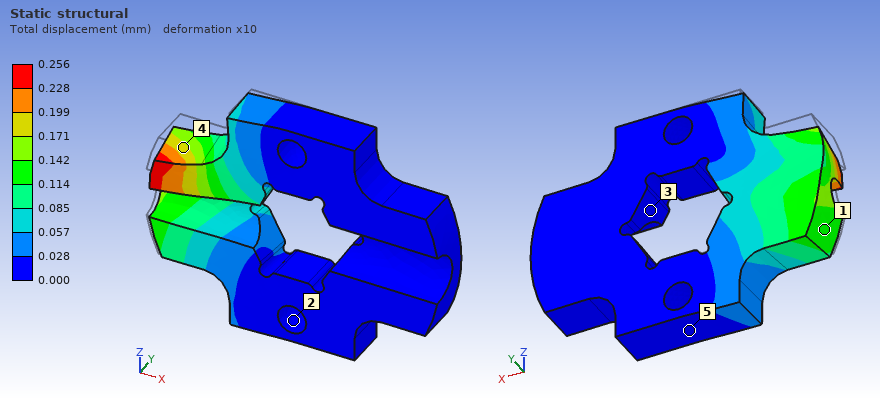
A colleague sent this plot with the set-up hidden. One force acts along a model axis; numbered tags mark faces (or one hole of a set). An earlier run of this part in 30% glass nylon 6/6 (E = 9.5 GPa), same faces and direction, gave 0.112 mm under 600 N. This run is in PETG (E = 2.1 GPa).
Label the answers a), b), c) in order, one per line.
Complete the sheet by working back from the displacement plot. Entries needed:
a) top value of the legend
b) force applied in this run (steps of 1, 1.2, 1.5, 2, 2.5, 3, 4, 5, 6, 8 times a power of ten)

a) 0.256 mm
b) 300 N
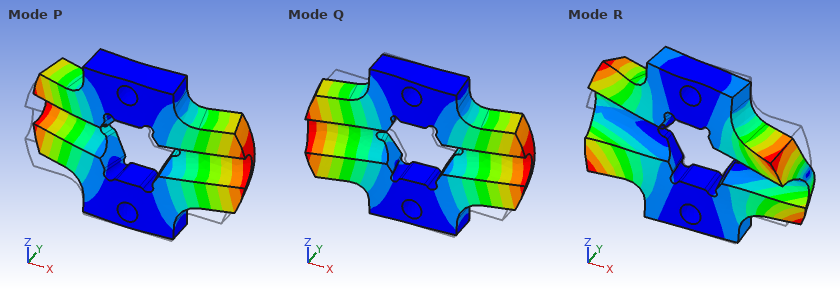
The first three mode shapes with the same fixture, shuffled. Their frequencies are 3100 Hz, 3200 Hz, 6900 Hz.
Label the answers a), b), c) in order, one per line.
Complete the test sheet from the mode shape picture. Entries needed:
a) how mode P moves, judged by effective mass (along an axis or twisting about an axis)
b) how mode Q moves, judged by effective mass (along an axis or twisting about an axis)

a) along Y
b) twisting about Z
